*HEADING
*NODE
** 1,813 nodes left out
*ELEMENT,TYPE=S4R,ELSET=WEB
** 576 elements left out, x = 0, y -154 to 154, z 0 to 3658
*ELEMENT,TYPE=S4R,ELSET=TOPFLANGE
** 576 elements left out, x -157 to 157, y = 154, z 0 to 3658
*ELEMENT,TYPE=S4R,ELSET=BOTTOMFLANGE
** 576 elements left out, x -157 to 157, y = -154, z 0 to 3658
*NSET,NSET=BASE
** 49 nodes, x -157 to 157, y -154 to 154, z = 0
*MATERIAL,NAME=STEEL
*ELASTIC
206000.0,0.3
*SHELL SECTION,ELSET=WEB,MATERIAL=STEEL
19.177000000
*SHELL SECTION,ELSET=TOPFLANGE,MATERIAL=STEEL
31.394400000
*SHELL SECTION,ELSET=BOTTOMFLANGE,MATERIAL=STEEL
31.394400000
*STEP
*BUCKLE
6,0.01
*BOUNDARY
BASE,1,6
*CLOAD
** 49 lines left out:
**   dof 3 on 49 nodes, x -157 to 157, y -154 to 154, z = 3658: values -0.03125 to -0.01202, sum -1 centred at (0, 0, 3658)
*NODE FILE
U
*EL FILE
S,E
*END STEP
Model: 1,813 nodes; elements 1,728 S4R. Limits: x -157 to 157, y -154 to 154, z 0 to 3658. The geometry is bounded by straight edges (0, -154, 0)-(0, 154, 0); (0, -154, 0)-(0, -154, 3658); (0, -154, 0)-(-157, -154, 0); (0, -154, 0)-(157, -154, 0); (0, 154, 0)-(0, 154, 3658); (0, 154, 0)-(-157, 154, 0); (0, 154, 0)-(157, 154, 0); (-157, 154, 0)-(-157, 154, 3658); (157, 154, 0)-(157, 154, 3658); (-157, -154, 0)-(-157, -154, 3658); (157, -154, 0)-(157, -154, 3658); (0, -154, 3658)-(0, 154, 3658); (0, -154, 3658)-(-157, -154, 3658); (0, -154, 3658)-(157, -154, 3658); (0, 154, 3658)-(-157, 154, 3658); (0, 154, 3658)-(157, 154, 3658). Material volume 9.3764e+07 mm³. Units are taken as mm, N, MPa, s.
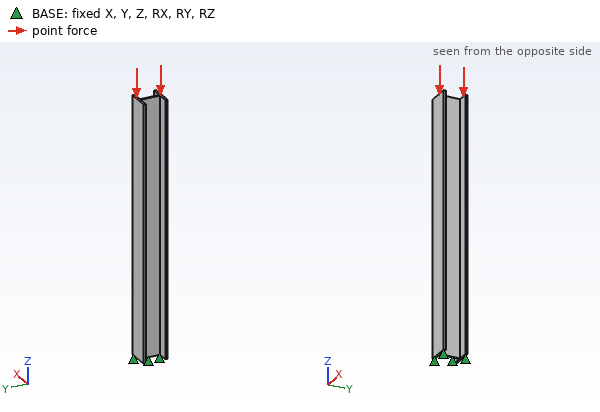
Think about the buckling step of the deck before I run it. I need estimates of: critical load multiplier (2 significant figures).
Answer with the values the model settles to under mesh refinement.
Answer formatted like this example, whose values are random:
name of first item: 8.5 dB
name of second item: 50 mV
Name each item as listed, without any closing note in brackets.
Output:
critical load multiplier: 6.1e+06
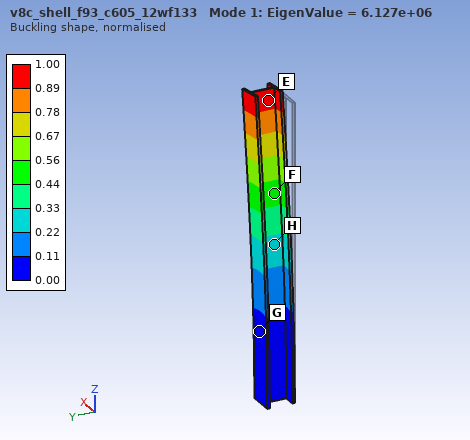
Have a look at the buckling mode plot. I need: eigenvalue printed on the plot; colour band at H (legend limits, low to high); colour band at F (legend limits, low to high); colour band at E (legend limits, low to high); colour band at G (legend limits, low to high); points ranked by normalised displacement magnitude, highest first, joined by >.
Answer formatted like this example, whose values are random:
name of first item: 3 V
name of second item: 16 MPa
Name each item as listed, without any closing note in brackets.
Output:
eigenvalue printed on the plot: 6.127e+06
colour band at H: 0.22 to 0.33
colour band at F: 0.44 to 0.56
colour band at E: 0.89 to 1.00
colour band at G: 0.00 to 0.11
points ranked by normalised displacement magnitude, highest first, joined by >: E > F > H > G
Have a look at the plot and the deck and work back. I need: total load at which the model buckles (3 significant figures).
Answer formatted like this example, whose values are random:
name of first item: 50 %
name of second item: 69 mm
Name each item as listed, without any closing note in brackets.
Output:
total load at which the model buckles: 6.13e+06 N
